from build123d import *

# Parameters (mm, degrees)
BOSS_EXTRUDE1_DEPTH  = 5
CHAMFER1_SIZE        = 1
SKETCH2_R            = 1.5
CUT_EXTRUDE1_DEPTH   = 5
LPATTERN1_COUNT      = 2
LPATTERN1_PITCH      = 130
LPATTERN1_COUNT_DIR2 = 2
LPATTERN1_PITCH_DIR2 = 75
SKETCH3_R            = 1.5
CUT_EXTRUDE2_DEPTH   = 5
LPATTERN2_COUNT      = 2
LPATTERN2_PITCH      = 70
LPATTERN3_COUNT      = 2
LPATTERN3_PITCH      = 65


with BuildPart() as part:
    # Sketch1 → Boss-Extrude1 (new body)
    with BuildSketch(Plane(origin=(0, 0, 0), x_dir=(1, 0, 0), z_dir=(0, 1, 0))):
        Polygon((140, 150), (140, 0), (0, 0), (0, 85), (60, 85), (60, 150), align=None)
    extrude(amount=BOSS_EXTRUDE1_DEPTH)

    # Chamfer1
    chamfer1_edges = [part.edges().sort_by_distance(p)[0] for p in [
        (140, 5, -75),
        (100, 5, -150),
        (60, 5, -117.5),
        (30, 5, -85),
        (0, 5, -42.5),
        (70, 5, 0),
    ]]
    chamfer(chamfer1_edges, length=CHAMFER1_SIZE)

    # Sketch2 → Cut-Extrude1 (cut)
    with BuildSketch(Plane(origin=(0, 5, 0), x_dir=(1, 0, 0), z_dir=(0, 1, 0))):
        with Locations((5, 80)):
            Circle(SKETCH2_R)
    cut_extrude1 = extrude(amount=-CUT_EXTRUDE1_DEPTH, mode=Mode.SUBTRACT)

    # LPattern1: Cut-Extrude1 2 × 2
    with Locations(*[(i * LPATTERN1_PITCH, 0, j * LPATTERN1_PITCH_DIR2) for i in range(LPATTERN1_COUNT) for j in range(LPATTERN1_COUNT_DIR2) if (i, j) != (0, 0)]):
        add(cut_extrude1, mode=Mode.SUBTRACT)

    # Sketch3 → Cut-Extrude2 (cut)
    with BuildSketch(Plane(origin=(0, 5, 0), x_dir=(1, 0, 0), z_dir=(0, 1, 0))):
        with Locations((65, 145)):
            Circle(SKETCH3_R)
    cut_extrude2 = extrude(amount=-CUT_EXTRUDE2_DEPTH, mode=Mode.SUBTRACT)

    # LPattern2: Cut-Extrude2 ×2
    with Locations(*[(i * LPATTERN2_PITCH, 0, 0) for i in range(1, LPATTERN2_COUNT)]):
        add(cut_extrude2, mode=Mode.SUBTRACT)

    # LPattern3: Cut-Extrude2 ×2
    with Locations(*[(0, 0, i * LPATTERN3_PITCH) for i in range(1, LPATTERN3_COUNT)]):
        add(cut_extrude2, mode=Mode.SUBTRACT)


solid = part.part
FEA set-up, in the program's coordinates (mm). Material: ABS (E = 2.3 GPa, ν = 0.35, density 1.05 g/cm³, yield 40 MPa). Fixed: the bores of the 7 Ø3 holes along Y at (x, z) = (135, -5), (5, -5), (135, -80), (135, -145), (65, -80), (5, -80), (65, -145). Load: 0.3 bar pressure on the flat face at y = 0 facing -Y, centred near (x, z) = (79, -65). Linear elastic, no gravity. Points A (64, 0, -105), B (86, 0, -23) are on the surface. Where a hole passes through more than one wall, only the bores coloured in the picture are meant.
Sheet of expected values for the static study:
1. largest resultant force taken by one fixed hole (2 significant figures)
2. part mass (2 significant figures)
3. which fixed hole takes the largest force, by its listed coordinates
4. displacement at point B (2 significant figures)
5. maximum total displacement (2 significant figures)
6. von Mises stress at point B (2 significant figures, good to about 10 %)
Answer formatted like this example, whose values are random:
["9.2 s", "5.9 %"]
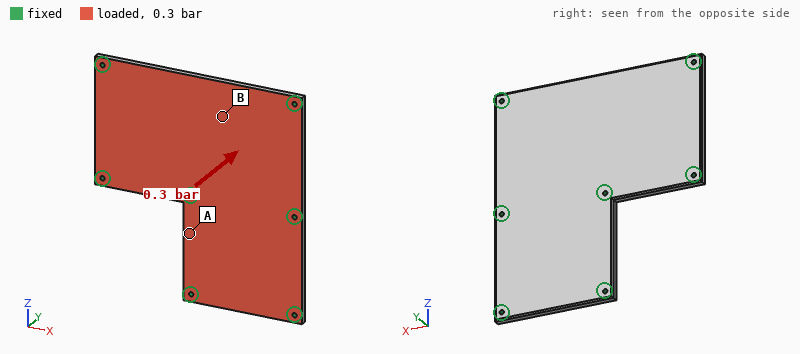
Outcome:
["160 N", "89 g", "(65, -80)", "0.82 mm", "1.2 mm", "3.7 MPa"]
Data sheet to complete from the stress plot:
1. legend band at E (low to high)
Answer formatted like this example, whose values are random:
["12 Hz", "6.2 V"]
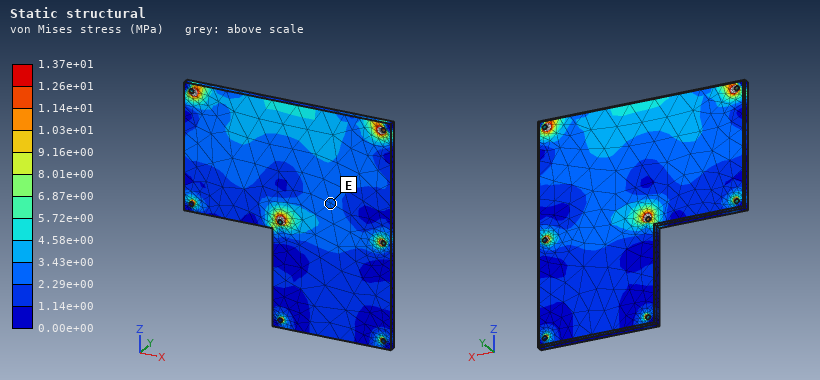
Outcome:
["2.29e+00 to 3.43e+00 MPa"]
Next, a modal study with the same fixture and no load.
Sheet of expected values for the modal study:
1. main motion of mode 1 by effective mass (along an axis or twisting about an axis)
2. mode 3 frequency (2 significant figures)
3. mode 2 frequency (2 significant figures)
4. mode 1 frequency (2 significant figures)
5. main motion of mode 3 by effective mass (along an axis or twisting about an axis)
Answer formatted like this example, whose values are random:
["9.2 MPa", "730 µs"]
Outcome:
["along Y", "1000 Hz", "950 Hz", "470 Hz", "along Y"]
